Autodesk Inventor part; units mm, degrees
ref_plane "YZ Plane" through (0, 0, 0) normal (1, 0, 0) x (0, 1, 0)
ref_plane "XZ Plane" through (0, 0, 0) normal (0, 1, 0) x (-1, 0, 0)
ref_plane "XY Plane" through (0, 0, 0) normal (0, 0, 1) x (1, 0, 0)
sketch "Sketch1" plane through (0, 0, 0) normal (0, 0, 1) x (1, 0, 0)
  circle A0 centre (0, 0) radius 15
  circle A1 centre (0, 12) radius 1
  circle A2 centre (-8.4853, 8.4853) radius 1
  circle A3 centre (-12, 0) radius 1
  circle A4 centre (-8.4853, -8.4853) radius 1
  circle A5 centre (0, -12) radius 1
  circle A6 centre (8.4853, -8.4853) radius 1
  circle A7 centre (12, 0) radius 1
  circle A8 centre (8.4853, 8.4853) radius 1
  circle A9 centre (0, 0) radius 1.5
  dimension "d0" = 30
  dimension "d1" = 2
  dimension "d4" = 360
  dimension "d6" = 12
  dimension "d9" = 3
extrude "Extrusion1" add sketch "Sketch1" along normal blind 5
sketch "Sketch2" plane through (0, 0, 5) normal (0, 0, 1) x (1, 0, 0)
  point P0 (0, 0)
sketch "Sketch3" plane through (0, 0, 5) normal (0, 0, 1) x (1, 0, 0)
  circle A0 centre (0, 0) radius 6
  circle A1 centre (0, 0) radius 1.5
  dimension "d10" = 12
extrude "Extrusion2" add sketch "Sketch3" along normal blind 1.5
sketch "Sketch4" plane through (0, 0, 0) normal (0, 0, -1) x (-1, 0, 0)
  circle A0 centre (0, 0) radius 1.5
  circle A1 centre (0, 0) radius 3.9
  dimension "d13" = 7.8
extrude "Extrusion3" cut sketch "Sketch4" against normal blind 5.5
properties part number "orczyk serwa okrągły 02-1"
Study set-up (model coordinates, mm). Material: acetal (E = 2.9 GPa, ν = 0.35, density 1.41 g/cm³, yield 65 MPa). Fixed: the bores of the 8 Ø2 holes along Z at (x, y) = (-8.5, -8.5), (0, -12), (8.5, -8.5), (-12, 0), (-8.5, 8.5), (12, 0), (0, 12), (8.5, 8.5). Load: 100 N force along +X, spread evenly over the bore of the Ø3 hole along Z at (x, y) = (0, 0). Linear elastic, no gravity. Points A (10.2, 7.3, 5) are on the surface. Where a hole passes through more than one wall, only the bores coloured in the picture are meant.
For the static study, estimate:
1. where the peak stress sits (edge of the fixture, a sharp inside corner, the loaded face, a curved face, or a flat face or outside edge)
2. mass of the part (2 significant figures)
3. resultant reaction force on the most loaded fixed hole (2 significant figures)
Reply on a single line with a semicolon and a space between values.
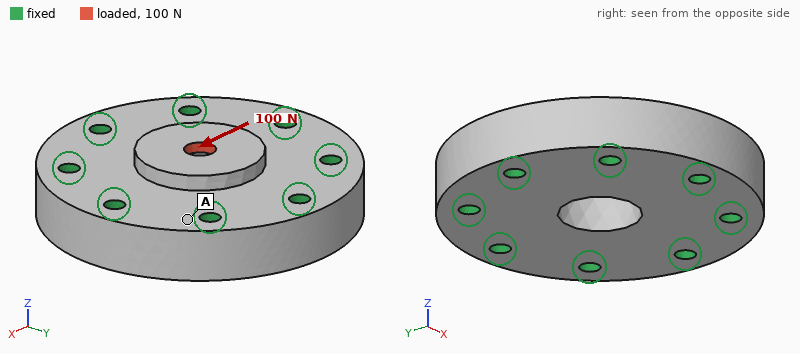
the loaded face; 4.7 g; 22 N
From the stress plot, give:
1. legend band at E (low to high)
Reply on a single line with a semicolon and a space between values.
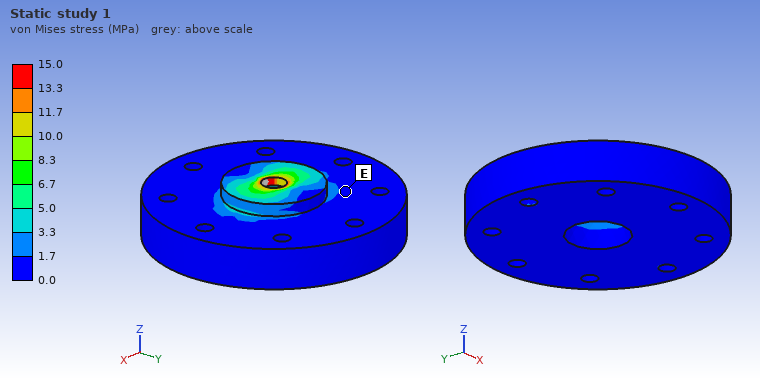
0.0 to 1.7 MPa
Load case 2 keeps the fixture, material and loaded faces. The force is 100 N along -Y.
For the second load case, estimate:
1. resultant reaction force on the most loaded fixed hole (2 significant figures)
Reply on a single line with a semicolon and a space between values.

22 N
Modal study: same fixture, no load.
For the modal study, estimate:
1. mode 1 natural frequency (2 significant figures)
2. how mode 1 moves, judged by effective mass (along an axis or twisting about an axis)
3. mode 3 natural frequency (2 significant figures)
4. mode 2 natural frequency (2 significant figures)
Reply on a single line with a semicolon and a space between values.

18 kHz; along Z; 26 kHz; 26 kHz
